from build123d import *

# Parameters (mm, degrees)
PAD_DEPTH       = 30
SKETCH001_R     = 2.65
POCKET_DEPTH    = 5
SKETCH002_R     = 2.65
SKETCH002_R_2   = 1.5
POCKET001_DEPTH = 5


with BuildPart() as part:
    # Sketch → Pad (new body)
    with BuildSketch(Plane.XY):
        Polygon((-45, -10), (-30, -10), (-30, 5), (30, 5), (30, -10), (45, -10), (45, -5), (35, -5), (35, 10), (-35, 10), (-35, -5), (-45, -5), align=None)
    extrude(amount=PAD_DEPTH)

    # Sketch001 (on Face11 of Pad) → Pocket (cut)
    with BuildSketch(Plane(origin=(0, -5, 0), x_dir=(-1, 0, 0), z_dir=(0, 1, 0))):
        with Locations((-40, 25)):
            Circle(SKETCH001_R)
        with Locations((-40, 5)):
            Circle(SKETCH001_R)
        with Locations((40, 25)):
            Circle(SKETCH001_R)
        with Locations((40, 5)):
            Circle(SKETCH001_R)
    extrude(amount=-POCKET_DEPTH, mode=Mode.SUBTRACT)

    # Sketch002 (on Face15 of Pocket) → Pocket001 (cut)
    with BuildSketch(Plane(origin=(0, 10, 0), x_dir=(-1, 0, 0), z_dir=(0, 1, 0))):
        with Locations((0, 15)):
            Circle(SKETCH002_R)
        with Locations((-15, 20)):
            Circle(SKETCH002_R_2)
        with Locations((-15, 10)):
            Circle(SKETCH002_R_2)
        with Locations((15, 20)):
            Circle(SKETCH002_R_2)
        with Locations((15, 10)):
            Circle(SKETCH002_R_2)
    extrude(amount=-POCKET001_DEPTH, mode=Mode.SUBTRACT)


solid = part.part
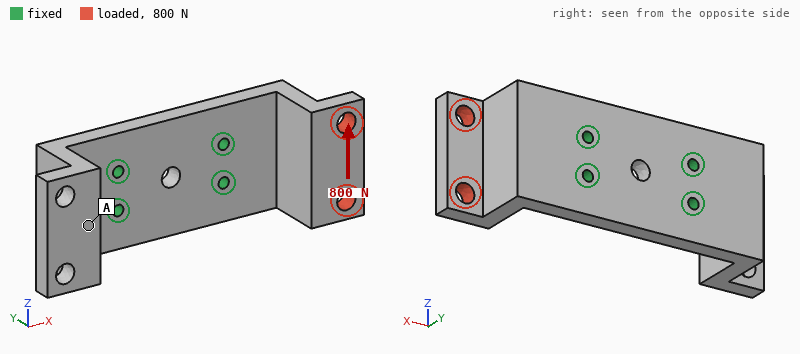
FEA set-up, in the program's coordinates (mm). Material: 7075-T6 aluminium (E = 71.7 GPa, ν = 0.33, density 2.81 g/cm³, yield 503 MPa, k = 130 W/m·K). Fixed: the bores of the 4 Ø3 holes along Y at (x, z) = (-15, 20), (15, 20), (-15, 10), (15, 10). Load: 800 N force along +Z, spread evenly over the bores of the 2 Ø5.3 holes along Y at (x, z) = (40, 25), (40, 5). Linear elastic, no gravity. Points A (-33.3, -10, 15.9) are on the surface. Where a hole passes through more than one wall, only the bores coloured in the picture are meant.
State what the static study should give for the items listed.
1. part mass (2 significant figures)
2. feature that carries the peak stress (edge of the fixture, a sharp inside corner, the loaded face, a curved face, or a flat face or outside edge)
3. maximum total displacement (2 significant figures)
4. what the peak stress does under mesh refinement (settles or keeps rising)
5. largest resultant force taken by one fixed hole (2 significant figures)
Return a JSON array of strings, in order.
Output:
["49 g", "edge of the fixture", "98 µm", "keeps rising", "1.3 kN"]
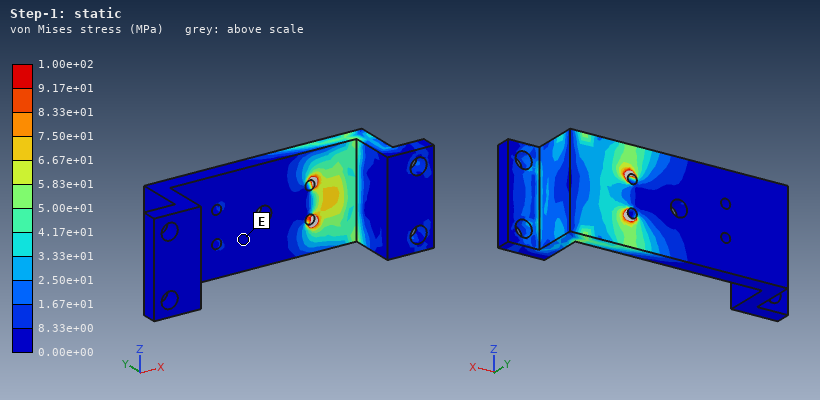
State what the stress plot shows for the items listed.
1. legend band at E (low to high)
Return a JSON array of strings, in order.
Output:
["0.00e+00 to 8.33e+00 MPa"]
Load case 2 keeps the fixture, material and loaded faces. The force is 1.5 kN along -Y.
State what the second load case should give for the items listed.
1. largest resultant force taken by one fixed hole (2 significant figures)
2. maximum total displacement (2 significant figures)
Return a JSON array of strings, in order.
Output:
["880 N", "0.67 mm"]
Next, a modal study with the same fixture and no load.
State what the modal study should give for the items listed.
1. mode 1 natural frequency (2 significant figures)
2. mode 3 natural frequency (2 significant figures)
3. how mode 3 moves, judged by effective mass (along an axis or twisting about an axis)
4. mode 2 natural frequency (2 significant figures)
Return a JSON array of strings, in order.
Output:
["2900 Hz", "5300 Hz", "twisting about Y", "2900 Hz"]
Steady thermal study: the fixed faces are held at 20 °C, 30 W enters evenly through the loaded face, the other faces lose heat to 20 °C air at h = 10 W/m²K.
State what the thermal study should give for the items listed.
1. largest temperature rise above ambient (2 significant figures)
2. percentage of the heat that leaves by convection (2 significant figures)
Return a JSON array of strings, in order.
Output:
["62 K", "3.6 %"]
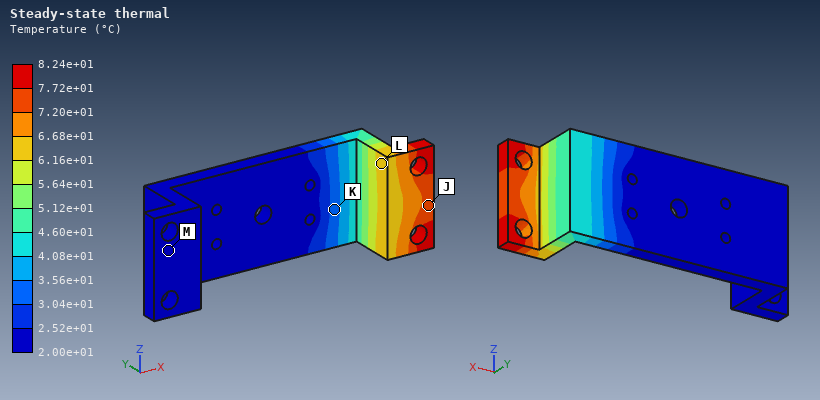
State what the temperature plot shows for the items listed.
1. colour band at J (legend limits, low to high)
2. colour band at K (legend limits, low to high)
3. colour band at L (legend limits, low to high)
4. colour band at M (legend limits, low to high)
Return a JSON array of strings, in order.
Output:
["7.20e+01 to 7.72e+01 °C", "3.04e+01 to 3.56e+01 °C", "6.16e+01 to 6.68e+01 °C", "2.00e+01 to 2.52e+01 °C"]
